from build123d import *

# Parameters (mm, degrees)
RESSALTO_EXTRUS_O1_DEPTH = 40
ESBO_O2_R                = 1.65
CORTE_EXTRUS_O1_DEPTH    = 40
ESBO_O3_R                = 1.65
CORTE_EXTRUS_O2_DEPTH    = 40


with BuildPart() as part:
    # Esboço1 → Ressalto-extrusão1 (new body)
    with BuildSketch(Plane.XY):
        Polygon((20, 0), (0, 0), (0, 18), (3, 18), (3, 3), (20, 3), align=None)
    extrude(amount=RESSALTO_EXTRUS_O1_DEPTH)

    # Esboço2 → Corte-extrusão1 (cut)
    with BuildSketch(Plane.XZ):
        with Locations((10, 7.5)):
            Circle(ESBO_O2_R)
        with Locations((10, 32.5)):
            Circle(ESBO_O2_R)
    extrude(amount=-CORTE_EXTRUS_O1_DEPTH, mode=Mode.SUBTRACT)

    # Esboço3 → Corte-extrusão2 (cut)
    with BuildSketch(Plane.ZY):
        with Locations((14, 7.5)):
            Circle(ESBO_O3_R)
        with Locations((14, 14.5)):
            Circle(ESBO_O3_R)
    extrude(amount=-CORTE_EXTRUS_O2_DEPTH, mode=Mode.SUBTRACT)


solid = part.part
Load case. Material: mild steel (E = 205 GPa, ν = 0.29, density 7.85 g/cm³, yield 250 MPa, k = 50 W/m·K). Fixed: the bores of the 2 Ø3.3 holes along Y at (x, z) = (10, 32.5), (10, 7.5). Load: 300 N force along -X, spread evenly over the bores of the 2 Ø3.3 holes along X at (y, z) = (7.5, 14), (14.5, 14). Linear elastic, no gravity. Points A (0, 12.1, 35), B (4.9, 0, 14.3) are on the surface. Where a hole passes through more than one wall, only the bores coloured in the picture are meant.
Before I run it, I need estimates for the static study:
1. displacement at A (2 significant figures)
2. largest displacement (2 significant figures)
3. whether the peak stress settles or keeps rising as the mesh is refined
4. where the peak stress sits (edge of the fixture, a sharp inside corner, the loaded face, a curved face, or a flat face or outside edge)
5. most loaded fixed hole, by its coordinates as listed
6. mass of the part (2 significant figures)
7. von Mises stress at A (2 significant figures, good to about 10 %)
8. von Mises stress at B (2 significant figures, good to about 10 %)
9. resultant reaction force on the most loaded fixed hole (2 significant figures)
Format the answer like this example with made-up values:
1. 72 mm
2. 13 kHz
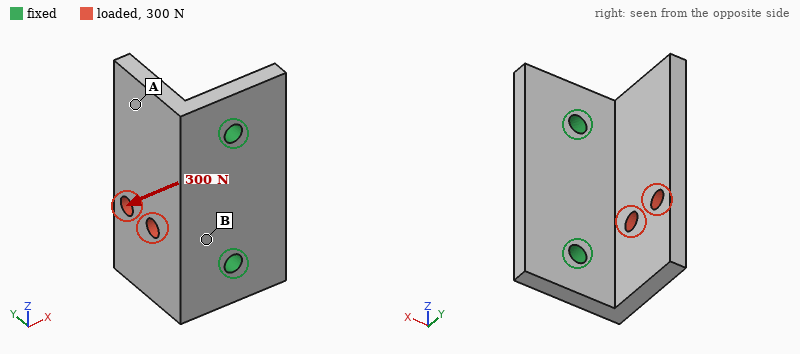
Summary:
1. 15 µm
2. 38 µm
3. keeps rising
4. edge of the fixture
5. (10, 7.5)
6. 32 g
7. 15 MPa
8. 44 MPa
9. 220 N
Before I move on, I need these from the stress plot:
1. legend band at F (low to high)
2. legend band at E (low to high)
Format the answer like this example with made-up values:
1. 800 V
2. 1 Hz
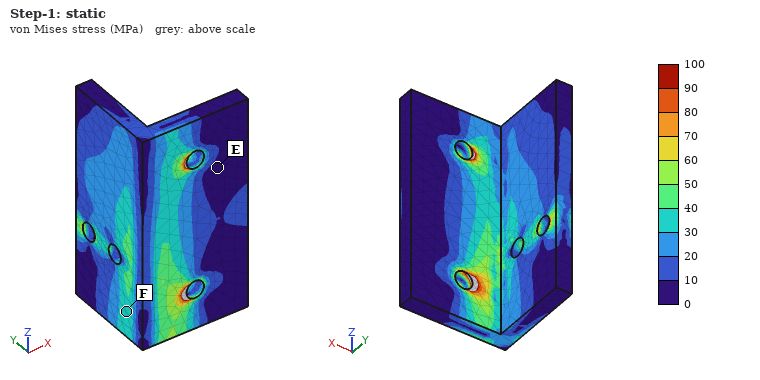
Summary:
1. 30 to 40 MPa
2. 0 to 10 MPa
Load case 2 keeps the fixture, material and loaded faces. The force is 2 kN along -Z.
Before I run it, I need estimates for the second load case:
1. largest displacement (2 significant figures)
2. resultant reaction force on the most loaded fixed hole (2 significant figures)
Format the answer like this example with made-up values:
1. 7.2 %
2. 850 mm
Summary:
1. 37 µm
2. 1.4 kN
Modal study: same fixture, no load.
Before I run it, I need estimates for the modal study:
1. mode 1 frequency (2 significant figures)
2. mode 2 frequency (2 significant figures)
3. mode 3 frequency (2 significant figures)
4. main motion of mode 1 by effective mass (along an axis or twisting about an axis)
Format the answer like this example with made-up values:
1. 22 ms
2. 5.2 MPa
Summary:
1. 5000 Hz
2. 8300 Hz
3. 14 kHz
4. along X
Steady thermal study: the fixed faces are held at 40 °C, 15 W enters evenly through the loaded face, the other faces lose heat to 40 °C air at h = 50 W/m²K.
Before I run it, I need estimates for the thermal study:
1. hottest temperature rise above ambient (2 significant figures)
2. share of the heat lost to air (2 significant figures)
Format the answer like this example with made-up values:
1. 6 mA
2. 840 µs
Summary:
1. 64 K
2. 21 %
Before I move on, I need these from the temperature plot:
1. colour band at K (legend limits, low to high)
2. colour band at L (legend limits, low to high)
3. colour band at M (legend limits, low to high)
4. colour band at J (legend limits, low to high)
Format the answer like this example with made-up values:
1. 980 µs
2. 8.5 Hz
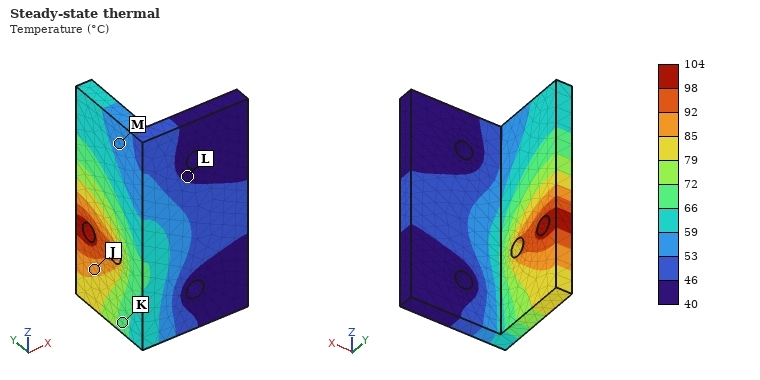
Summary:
1. 66 to 72 °C
2. 40 to 46 °C
3. 53 to 59 °C
4. 85 to 92 °C
